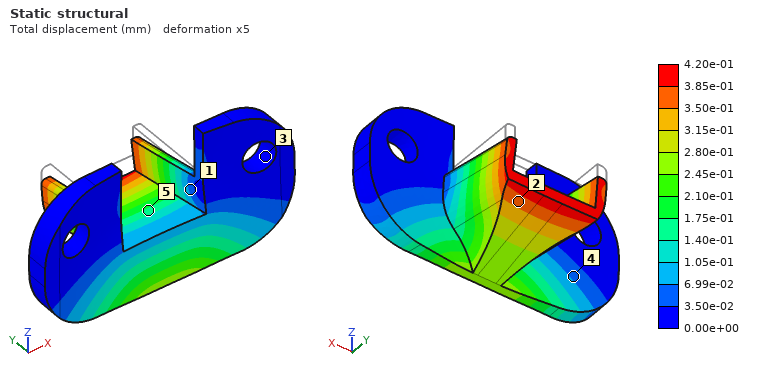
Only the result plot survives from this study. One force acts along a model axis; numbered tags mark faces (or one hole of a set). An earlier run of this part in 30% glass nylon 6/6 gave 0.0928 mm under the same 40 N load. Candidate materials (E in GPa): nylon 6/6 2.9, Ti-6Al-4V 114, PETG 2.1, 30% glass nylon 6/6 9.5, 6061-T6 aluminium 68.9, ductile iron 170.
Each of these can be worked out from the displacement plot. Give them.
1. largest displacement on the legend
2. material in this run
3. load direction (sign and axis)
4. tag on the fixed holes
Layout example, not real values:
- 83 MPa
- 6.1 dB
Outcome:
- 4.20e-01 mm
- PETG
- -Z
- 3
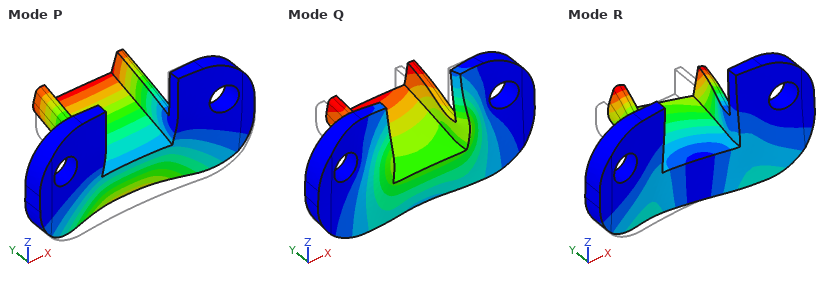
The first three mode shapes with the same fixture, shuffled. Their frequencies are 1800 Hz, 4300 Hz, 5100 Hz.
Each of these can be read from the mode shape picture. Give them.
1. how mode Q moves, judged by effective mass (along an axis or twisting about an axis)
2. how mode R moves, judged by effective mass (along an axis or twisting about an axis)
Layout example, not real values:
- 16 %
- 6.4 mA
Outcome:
- along Y
- along X
